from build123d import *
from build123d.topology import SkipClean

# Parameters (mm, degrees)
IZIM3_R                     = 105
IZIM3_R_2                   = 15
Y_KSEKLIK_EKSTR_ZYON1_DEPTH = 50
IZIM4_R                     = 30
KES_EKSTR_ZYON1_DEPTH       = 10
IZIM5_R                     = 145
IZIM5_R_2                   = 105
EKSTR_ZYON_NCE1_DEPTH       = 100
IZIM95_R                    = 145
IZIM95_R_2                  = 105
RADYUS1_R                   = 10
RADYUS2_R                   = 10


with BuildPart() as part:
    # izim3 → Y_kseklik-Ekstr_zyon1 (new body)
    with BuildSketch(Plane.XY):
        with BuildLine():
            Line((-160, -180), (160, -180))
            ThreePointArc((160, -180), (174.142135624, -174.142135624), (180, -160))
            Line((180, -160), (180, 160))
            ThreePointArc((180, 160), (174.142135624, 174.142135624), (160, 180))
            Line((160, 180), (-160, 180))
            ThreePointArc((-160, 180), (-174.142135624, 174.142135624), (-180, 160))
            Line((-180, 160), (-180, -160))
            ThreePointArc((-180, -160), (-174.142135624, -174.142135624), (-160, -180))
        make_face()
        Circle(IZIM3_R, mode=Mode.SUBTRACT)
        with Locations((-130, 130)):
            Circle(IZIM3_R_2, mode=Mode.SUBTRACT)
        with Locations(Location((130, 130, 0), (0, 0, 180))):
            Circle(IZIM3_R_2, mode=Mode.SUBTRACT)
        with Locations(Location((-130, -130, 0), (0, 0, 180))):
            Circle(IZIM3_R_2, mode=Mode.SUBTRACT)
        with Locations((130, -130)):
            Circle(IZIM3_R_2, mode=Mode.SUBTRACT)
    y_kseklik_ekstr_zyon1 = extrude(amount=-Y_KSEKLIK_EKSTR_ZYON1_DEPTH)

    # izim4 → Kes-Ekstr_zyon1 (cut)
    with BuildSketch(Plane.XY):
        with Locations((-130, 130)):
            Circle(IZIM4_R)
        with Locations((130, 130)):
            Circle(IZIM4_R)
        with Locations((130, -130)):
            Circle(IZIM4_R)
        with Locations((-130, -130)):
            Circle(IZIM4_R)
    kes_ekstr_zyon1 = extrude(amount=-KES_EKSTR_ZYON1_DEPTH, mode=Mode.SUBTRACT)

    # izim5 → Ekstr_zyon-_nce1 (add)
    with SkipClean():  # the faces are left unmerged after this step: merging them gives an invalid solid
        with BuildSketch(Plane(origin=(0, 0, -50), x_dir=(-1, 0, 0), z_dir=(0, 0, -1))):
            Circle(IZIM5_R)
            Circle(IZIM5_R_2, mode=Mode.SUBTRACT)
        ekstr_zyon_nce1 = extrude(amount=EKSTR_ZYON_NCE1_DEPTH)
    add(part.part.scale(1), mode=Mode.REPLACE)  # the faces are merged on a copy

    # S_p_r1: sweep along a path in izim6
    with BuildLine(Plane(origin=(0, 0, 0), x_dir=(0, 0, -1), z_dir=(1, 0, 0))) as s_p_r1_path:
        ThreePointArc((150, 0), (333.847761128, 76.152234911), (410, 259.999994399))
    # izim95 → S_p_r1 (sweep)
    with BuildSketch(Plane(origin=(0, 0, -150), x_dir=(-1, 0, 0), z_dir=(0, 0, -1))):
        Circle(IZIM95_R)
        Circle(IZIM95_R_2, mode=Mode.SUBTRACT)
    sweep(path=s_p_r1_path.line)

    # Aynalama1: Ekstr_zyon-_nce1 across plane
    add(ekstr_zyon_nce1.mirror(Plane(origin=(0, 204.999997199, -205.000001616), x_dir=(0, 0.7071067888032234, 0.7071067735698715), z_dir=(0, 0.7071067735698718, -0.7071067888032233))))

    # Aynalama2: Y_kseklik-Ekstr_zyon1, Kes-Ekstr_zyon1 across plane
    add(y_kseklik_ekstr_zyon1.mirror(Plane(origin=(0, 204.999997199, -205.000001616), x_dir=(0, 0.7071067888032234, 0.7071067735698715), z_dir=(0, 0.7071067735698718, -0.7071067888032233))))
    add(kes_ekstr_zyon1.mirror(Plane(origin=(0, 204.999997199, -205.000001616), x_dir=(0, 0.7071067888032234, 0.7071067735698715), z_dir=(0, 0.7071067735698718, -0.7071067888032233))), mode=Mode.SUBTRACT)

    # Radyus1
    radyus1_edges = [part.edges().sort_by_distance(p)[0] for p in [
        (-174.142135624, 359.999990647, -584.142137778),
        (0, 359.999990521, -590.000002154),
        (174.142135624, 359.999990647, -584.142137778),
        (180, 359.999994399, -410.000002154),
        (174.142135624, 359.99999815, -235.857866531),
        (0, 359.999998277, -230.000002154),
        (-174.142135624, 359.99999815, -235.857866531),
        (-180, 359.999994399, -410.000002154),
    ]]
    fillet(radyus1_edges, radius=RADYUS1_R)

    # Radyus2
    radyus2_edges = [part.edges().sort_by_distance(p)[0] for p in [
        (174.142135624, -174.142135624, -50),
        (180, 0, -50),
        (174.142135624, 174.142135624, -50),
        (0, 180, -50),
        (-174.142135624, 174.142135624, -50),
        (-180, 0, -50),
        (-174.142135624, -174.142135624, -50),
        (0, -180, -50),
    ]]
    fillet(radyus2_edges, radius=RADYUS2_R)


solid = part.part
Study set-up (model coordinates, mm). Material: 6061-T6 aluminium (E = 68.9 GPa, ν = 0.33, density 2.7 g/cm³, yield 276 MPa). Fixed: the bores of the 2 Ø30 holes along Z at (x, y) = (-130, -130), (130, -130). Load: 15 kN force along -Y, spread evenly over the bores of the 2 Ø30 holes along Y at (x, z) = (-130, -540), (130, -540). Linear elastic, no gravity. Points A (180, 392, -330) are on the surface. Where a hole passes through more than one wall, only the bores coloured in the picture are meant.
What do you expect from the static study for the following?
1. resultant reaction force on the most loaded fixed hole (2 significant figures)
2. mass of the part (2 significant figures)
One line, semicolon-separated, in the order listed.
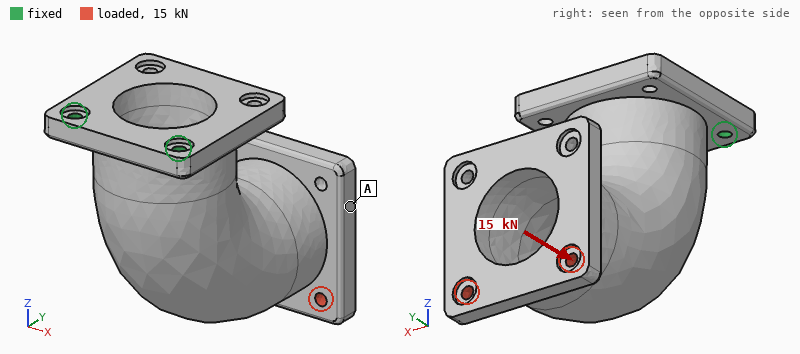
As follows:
7.6 kN; 76 kg
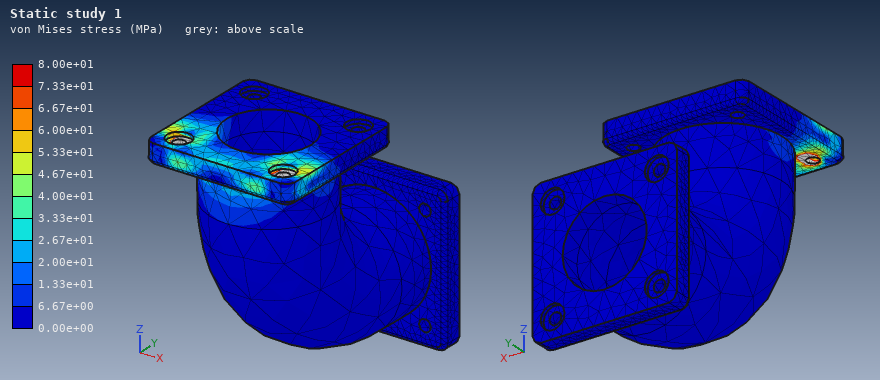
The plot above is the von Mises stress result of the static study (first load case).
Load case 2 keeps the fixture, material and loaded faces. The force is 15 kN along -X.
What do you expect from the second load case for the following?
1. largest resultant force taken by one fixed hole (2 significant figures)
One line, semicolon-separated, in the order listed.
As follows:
42 kN
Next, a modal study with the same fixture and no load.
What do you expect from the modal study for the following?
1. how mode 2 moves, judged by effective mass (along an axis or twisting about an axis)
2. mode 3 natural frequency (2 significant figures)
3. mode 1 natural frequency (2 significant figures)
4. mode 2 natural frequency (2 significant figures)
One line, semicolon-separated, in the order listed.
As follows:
along X; 540 Hz; 68 Hz; 220 Hz
